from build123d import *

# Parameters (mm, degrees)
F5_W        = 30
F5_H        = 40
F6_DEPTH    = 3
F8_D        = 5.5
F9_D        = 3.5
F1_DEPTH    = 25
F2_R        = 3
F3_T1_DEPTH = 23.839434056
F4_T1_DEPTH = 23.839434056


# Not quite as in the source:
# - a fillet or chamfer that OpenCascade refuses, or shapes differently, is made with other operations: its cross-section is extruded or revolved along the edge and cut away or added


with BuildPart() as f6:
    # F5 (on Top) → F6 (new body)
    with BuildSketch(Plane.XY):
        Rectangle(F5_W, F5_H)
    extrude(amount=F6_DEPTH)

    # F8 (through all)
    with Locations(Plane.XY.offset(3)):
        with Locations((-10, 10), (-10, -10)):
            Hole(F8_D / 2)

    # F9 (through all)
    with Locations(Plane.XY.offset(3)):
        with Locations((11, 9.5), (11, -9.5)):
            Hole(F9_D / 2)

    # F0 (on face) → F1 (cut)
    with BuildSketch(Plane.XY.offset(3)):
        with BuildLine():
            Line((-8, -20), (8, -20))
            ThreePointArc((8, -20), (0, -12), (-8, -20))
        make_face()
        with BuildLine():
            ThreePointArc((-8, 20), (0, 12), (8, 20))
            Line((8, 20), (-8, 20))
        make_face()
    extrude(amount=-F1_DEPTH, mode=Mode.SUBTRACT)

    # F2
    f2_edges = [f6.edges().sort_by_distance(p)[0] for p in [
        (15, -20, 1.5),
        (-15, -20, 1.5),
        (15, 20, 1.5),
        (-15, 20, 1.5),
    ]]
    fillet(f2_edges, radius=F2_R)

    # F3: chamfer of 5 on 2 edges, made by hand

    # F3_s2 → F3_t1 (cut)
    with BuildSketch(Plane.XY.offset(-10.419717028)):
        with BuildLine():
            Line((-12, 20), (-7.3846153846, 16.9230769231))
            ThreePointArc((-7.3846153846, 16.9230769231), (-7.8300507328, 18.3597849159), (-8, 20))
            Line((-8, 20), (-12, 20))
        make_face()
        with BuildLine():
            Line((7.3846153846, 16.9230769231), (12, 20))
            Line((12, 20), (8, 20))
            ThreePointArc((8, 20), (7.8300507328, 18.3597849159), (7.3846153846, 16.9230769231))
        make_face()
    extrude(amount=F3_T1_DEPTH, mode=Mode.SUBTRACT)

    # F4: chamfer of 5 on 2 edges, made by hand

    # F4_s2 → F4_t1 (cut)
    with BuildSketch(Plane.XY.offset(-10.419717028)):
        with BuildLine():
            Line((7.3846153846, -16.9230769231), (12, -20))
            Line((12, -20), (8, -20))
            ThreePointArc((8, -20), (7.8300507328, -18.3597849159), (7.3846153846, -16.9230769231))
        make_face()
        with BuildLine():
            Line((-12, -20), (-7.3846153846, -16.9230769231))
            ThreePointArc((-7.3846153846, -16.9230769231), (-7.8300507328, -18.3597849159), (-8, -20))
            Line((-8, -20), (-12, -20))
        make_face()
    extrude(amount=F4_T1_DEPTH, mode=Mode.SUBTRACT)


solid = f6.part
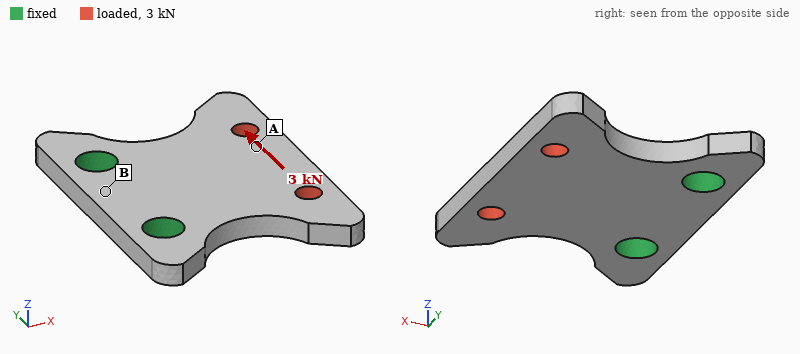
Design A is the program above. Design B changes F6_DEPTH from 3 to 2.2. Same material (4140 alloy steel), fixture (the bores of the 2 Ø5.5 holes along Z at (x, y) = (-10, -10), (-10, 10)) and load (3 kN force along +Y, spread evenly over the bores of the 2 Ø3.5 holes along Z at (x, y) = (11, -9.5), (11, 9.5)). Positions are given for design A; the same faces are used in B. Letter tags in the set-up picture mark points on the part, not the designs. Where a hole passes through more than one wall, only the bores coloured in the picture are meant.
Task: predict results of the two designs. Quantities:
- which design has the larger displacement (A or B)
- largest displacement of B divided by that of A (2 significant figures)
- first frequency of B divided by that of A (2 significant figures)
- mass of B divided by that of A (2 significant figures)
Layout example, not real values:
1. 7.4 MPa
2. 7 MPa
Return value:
1. B
2. 1.4
3. 0.75
4. 0.73
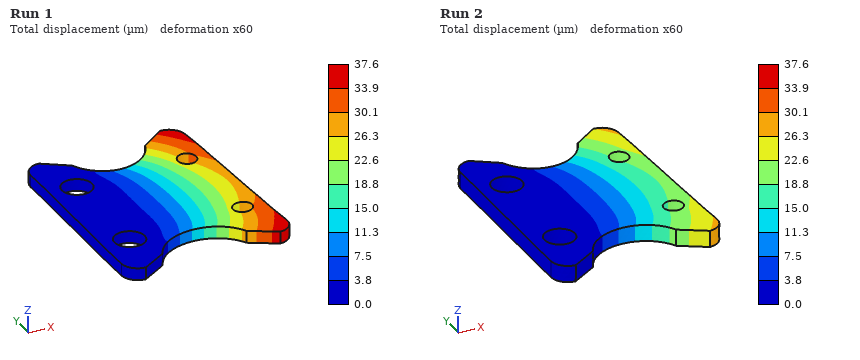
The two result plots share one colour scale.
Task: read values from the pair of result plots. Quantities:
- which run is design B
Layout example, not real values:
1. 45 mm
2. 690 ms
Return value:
1. Run 1
